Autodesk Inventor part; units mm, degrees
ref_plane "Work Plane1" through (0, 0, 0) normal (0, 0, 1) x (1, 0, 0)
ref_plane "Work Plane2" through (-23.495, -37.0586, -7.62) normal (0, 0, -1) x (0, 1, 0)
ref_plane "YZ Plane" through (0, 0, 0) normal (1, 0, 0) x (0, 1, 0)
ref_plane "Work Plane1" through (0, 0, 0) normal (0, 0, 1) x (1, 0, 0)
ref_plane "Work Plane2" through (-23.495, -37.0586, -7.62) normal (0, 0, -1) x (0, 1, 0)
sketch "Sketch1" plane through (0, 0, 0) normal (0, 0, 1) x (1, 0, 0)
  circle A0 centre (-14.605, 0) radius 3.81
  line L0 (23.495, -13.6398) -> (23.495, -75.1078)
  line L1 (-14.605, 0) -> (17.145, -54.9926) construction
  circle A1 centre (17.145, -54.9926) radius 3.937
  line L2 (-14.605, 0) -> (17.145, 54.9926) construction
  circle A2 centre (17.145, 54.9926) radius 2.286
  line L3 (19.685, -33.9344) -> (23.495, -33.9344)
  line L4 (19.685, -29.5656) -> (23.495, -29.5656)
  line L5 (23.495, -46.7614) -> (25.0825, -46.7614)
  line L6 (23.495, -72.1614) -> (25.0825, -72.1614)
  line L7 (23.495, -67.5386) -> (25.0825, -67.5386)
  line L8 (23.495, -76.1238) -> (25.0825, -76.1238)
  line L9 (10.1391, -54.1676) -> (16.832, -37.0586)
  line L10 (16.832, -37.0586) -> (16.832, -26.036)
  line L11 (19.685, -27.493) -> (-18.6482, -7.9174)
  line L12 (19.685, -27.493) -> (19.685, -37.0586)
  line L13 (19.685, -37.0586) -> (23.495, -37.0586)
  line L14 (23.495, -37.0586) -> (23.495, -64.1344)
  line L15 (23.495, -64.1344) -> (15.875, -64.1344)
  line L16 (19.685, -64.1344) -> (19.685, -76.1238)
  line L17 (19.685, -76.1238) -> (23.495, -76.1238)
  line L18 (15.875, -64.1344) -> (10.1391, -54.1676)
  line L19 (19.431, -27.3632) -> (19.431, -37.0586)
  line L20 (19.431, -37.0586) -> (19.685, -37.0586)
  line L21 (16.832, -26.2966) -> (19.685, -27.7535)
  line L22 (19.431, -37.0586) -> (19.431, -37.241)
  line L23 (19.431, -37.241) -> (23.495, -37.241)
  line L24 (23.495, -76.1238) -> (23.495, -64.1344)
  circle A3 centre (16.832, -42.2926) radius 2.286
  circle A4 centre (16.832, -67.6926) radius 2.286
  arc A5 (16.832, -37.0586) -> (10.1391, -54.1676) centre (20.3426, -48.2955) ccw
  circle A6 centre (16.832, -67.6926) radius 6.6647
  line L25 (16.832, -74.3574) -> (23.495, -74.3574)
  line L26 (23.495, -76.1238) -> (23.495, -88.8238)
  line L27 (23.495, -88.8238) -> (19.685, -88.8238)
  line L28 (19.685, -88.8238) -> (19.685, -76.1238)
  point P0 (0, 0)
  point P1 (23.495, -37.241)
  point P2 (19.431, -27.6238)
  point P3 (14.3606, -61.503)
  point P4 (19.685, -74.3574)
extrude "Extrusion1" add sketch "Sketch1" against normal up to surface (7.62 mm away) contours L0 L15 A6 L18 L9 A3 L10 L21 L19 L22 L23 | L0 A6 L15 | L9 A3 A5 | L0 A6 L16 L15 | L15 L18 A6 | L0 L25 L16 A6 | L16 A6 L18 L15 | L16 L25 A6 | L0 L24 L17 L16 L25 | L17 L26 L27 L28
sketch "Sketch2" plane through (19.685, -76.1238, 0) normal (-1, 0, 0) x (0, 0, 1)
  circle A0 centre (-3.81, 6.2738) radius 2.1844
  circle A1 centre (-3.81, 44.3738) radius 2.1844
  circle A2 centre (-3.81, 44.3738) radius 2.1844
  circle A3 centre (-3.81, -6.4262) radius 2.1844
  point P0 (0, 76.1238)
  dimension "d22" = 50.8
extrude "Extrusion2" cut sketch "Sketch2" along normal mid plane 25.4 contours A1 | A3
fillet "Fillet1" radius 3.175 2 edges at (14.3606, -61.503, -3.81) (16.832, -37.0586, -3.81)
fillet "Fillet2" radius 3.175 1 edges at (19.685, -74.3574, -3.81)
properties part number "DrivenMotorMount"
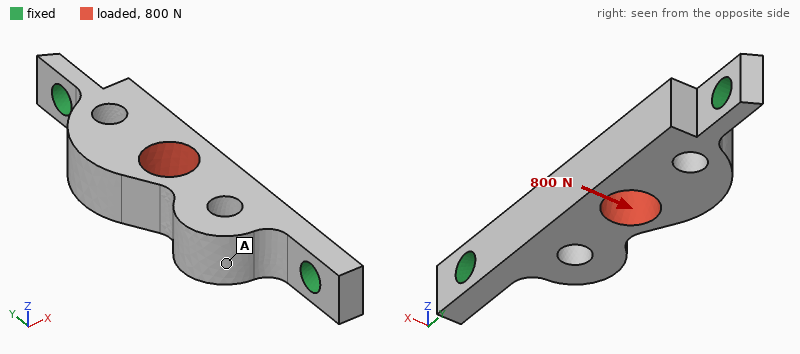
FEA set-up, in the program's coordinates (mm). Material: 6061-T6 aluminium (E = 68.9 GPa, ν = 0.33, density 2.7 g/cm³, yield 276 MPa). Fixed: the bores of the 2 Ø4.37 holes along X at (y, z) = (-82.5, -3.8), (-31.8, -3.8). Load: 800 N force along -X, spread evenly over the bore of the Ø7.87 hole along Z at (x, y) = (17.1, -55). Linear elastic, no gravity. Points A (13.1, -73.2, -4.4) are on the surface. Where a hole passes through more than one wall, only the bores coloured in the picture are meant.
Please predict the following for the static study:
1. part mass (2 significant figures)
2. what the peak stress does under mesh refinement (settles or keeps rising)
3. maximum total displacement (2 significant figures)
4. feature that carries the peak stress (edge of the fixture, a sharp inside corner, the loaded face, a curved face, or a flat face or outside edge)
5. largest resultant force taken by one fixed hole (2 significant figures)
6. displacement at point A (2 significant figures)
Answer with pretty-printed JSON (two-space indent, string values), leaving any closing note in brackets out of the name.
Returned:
{
  "part mass": "9.4 g",
  "what the peak stress does under mesh refinement": "keeps rising",
  "maximum total displacement": "37 µm",
  "feature that carries the peak stress": "edge of the fixture",
  "largest resultant force taken by one fixed hole": "450 N",
  "displacement at point A": "19 µm"
}
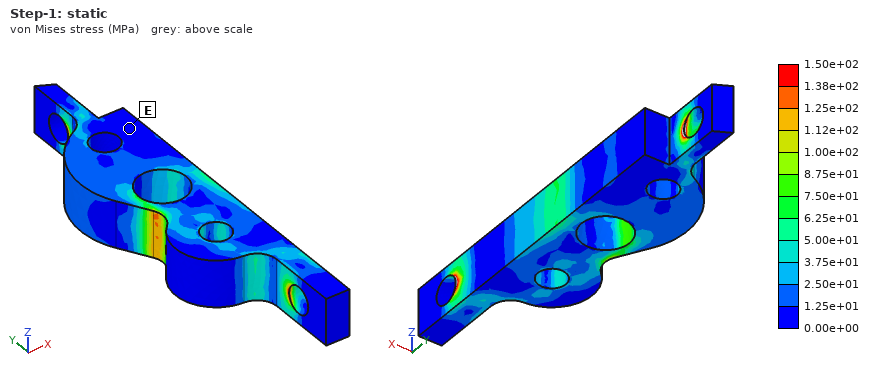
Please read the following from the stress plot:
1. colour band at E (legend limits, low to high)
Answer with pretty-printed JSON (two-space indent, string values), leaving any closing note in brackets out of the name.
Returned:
{
  "colour band at E": "0.00e+00 to 1.25e+01 MPa"
}
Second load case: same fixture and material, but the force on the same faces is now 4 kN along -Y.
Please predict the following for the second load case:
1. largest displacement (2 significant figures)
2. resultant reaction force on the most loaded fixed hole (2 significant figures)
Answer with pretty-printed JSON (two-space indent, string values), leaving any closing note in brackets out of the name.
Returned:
{
  "largest displacement": "25 µm",
  "resultant reaction force on the most loaded fixed hole": "2.1 kN"
}
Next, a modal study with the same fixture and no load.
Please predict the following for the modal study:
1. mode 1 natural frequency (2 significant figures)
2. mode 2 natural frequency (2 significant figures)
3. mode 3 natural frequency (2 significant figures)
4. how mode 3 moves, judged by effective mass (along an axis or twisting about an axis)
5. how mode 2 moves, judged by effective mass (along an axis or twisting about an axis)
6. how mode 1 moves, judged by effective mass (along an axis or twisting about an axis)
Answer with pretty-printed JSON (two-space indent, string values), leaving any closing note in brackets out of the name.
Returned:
{
  "mode 1 natural frequency": "7700 Hz",
  "mode 2 natural frequency": "11 kHz",
  "mode 3 natural frequency": "12 kHz",
  "how mode 3 moves, judged by effective mass": "along Z",
  "how mode 2 moves, judged by effective mass": "along X",
  "how mode 1 moves, judged by effective mass": "along Z"
}
